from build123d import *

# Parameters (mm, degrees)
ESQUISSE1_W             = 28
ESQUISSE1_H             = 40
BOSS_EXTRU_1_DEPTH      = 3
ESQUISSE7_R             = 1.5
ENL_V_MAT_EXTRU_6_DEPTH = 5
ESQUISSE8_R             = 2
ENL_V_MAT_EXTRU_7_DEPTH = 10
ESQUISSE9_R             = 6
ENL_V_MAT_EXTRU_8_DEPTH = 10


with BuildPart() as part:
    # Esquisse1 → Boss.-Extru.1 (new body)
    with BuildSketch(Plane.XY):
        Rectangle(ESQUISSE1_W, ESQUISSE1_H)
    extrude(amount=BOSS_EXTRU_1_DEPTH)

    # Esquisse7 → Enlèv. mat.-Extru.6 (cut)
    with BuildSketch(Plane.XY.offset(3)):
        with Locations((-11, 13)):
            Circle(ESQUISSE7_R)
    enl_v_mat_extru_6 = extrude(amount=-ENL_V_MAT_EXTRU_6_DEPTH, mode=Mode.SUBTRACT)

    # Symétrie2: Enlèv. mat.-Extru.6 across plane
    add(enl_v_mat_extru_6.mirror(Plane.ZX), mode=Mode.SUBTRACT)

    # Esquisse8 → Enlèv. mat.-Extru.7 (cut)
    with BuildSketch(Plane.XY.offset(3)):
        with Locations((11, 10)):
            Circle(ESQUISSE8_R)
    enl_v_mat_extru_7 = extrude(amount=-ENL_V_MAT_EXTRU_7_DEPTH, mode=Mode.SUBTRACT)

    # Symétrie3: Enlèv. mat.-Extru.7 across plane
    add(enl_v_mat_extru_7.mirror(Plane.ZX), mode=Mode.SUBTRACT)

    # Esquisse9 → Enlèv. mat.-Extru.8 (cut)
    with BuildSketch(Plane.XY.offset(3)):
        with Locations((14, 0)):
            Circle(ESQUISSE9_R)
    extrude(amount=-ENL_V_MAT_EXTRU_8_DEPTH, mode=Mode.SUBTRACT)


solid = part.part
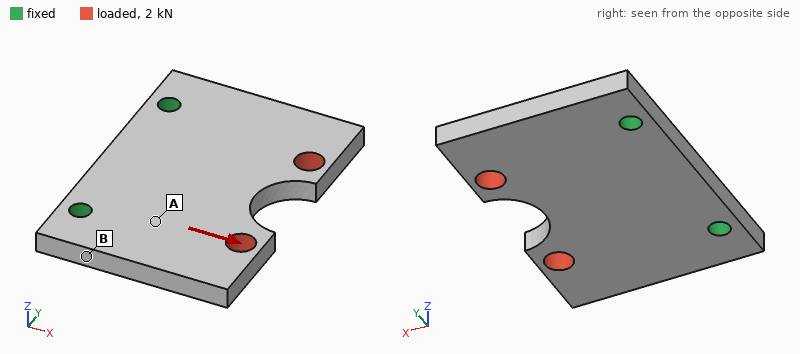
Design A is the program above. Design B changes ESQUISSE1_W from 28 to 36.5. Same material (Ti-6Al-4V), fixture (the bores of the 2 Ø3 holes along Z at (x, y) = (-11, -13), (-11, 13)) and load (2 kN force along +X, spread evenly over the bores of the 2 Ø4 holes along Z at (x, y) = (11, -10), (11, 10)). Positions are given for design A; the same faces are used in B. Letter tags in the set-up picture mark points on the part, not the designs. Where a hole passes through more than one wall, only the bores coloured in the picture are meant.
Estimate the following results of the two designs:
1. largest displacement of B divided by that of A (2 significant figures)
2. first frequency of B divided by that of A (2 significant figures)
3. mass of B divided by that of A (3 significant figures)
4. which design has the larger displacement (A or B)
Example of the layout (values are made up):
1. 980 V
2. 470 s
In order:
1. 0.71
2. 0.78
3. 1.29
4. A
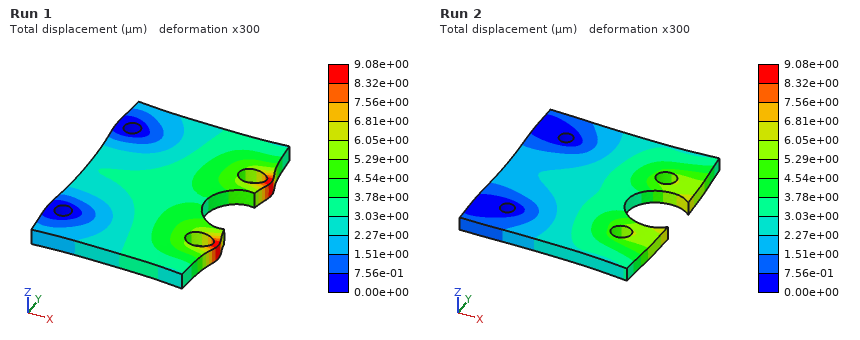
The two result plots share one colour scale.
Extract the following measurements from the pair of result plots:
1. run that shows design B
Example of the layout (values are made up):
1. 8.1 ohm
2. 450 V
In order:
1. Run 2
